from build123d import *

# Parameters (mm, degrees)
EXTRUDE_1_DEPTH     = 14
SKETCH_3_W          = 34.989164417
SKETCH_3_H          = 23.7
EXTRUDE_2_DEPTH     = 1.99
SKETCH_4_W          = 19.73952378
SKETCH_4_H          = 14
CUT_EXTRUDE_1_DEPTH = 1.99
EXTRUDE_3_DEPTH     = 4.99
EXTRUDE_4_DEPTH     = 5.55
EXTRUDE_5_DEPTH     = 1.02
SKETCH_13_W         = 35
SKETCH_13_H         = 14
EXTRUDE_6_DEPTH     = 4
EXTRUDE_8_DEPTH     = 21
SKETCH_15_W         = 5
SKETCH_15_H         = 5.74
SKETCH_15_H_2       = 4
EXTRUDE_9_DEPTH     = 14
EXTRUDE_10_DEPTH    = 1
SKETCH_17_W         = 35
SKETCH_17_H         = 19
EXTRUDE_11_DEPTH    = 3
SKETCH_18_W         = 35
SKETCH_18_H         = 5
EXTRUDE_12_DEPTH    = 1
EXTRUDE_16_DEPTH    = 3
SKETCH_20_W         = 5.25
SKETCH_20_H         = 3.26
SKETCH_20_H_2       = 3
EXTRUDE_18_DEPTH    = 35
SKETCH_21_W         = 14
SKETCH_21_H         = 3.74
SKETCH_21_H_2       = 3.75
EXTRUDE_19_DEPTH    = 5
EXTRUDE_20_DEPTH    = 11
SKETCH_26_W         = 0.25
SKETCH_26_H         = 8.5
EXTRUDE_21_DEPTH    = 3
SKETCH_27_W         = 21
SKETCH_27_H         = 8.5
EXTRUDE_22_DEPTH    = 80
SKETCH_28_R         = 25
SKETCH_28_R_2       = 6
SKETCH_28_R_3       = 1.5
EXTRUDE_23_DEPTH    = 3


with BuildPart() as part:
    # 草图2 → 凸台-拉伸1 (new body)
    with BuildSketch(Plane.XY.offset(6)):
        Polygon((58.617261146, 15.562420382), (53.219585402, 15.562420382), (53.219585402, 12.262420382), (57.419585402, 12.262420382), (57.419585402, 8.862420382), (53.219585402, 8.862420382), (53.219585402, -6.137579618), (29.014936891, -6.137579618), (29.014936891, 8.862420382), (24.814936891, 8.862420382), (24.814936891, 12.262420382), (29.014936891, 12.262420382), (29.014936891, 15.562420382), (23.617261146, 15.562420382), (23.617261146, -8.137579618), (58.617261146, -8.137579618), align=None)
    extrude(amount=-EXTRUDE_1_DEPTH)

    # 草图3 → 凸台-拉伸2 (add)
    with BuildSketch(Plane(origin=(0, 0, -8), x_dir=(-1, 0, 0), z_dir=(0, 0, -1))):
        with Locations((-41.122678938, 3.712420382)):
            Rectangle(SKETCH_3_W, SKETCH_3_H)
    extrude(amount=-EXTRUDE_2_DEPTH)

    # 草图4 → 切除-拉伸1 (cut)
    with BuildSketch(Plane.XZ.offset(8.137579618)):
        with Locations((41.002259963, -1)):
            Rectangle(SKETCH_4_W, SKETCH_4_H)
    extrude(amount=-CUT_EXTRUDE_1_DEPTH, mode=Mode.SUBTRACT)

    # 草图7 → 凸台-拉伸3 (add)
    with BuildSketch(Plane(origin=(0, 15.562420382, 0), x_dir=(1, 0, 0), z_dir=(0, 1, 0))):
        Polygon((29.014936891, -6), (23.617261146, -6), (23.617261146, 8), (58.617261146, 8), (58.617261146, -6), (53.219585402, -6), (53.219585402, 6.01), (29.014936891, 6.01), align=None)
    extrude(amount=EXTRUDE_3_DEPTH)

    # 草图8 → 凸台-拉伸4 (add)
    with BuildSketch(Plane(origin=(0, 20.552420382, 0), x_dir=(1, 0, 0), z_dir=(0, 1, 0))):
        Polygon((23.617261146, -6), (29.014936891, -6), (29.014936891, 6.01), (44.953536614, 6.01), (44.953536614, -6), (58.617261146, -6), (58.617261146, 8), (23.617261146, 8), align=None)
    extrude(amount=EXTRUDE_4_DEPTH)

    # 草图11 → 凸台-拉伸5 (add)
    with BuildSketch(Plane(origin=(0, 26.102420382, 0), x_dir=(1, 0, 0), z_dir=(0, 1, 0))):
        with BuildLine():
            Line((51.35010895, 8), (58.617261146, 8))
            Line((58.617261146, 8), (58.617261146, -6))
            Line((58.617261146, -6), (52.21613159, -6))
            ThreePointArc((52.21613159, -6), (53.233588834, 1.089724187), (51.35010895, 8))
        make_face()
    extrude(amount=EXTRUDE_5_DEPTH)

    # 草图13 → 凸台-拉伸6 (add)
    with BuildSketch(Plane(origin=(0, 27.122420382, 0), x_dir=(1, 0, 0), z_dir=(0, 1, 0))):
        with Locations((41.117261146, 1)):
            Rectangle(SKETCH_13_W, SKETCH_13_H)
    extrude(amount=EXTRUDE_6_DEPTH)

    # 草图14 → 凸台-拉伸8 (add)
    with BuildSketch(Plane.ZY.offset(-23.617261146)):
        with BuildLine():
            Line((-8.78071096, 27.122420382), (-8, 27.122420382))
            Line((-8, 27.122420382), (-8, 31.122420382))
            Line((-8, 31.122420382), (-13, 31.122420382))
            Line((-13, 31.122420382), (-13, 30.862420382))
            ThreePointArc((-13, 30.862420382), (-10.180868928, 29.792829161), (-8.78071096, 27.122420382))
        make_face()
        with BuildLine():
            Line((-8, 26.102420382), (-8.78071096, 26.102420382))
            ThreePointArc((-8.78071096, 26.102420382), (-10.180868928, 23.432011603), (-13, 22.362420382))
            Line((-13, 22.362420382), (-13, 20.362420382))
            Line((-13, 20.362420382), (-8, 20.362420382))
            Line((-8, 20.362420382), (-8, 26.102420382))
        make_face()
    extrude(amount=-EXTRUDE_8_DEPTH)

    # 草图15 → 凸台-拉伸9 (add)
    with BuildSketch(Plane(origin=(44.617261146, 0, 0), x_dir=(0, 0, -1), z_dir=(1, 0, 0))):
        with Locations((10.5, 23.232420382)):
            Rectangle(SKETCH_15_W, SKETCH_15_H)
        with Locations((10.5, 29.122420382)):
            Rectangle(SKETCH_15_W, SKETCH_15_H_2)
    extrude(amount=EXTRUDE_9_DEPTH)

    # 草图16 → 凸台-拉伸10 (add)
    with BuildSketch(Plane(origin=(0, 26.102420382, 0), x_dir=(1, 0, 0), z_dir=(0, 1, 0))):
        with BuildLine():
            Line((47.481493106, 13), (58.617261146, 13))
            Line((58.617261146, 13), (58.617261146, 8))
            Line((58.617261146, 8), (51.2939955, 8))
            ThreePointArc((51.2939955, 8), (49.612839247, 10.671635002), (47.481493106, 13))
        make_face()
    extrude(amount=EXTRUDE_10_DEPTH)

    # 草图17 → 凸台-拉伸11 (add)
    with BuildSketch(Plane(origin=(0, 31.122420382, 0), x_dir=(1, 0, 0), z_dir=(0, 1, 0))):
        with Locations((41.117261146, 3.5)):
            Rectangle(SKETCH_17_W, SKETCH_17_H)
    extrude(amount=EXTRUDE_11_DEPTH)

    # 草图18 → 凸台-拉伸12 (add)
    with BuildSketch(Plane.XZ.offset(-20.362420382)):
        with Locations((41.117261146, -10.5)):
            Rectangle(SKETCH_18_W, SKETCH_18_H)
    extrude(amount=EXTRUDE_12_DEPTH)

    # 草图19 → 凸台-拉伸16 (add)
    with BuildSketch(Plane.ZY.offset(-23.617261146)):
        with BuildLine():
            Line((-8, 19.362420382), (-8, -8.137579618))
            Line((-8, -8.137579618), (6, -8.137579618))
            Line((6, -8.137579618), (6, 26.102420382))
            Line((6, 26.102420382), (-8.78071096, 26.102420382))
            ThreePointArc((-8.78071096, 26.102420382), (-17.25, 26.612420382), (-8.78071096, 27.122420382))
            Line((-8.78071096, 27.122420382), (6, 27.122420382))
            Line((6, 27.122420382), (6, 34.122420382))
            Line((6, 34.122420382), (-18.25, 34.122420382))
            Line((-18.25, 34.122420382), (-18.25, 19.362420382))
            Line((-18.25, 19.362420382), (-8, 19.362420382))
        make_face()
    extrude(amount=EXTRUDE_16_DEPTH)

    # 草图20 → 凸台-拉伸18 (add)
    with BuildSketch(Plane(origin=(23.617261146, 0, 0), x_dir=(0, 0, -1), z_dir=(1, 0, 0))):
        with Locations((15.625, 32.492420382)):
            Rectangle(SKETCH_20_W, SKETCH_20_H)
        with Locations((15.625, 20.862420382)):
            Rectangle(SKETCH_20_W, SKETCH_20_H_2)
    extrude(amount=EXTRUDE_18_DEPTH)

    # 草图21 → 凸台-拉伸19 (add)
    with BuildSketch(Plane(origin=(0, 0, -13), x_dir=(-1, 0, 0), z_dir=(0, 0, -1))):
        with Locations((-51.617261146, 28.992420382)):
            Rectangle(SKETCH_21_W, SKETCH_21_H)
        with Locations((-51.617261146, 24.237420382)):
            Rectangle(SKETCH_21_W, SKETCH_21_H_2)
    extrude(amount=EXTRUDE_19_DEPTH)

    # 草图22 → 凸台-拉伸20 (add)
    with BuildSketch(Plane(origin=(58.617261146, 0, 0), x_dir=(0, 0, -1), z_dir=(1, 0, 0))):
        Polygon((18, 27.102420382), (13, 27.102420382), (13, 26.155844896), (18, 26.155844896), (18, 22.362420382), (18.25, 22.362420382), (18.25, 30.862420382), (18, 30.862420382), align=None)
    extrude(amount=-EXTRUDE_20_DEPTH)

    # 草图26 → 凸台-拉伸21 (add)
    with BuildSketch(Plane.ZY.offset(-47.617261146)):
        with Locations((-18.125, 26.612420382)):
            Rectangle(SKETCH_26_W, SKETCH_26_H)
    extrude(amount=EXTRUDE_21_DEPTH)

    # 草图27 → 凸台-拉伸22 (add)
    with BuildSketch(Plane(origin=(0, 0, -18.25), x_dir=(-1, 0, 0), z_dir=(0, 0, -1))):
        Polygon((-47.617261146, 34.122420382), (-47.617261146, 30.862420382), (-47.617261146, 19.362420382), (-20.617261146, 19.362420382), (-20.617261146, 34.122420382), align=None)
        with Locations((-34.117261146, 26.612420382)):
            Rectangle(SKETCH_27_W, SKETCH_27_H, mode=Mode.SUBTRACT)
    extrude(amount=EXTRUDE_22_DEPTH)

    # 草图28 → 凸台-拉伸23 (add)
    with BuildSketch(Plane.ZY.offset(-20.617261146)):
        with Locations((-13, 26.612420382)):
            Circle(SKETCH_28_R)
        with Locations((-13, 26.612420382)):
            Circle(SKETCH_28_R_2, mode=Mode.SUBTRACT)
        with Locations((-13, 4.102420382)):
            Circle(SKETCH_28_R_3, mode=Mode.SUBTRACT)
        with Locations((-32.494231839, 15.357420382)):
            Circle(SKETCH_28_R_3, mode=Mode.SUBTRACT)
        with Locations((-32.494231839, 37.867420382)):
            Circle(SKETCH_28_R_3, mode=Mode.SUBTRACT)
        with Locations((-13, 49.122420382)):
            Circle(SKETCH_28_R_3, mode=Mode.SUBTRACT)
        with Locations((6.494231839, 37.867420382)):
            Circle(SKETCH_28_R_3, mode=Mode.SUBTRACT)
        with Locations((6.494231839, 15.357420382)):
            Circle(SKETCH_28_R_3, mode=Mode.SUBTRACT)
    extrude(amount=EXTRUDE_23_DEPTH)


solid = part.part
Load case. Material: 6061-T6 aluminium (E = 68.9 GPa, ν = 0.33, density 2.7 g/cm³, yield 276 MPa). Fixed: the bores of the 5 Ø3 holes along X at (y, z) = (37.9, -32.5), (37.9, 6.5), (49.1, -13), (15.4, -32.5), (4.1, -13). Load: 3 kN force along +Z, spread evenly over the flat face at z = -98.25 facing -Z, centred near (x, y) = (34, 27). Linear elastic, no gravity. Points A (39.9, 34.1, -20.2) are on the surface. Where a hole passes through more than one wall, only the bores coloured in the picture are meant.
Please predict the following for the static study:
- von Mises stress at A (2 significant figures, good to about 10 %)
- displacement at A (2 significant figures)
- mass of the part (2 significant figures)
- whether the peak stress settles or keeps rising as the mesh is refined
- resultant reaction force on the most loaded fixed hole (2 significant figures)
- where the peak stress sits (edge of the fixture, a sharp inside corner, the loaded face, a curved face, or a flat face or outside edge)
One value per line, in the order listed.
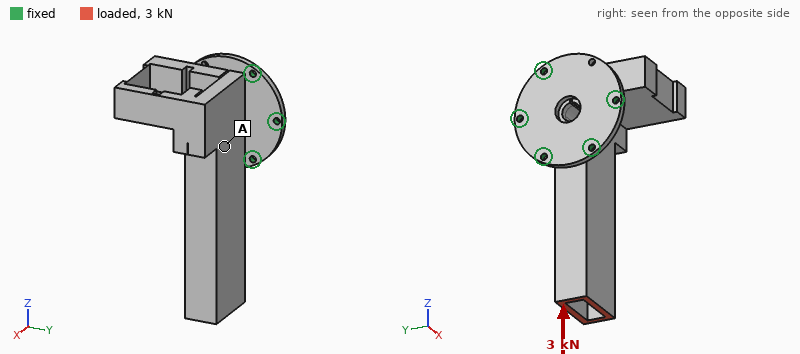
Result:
13 MPa
0.028 mm
110 g
keeps rising
1.2 kN
edge of the fixture
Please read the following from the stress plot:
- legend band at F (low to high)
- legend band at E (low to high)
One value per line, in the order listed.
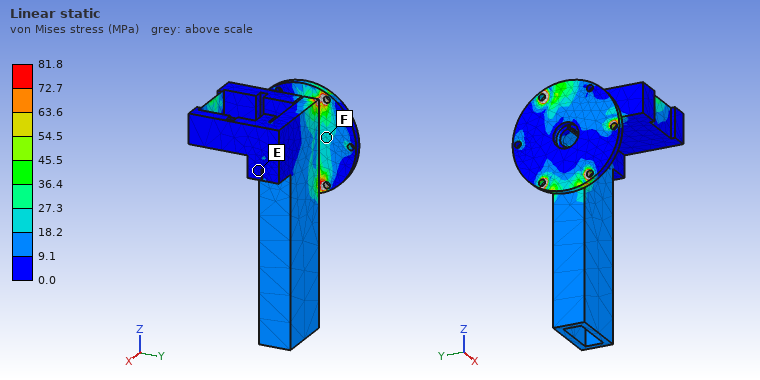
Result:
18.2 to 27.3 MPa
0.0 to 9.1 MPa
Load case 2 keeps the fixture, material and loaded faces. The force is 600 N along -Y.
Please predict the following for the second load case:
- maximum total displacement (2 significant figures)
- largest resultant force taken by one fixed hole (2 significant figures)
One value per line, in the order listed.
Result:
0.29 mm
1.1 kN
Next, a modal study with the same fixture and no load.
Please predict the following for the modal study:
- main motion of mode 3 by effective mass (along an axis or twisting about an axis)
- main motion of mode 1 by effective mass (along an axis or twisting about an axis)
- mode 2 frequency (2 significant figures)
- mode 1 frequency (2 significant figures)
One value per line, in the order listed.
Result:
along Y
along Y
2400 Hz
2000 Hz
